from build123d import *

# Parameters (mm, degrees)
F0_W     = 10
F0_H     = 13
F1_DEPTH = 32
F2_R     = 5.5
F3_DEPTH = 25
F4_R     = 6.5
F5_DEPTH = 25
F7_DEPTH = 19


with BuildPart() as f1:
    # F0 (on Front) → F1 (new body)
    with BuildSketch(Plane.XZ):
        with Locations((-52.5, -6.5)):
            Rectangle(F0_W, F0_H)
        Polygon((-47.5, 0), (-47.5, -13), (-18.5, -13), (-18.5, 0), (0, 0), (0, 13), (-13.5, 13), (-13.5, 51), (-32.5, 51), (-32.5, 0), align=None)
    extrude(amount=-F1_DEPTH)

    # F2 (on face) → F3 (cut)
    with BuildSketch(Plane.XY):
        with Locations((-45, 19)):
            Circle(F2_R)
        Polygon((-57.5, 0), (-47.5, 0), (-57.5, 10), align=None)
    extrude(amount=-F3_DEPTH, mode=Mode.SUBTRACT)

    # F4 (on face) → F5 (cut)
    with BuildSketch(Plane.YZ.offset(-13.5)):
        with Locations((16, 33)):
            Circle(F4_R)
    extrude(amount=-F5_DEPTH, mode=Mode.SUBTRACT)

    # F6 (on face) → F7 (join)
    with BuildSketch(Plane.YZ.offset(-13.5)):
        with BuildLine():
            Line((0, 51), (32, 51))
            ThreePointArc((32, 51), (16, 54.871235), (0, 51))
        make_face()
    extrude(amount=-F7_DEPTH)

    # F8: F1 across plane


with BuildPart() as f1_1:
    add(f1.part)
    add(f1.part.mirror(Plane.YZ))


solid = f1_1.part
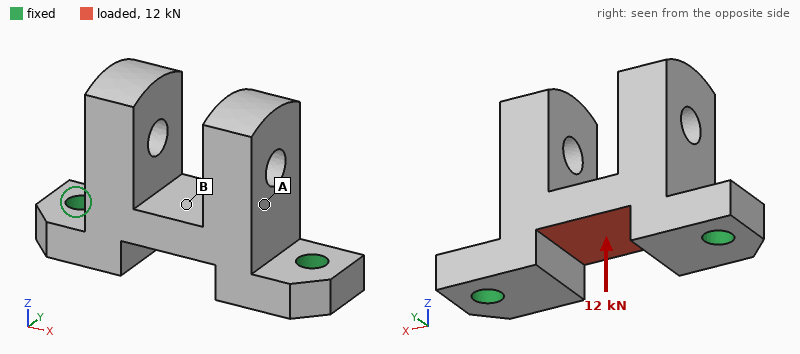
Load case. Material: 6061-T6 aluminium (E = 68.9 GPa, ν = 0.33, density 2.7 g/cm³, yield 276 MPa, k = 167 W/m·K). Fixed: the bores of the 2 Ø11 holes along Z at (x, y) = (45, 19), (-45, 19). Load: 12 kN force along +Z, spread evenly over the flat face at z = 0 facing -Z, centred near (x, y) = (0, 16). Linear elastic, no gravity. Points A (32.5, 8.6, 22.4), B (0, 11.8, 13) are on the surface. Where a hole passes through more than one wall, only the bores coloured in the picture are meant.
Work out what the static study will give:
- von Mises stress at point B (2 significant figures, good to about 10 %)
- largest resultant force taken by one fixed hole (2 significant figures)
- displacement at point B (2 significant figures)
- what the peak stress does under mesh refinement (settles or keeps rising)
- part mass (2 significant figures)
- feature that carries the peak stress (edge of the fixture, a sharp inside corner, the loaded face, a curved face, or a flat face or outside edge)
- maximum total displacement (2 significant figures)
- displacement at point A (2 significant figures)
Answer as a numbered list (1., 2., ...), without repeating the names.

1. 65 MPa
2. 9.4 kN
3. 52 µm
4. keeps rising
5. 270 g
6. edge of the fixture
7. 80 µm
8. 32 µm
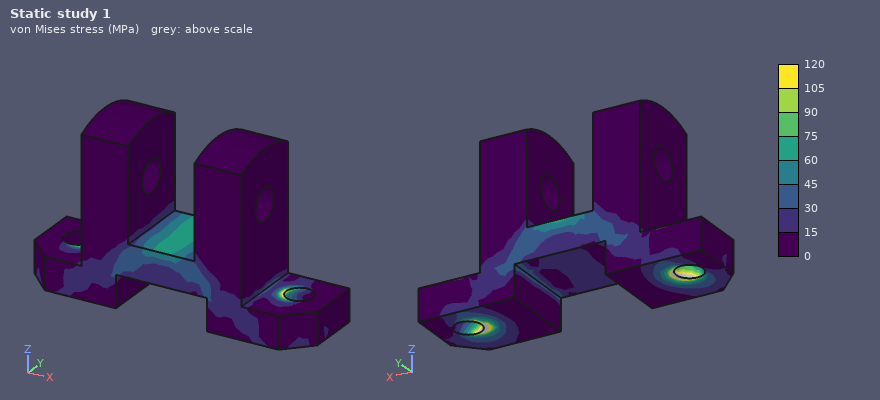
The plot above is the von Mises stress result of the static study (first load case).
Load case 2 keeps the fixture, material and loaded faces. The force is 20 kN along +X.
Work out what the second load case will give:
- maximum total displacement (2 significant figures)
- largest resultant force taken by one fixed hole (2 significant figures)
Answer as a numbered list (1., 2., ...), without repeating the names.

1. 49 µm
2. 10 kN
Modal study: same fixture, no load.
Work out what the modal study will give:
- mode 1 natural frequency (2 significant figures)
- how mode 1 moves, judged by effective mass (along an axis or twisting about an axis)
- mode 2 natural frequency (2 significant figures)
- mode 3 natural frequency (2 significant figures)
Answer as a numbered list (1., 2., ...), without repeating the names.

1. 2500 Hz
2. along Y
3. 3900 Hz
4. 4300 Hz
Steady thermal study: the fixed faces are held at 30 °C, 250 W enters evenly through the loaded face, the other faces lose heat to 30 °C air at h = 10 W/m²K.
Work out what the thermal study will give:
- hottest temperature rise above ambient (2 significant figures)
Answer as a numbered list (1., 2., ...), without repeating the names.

1. 66 K
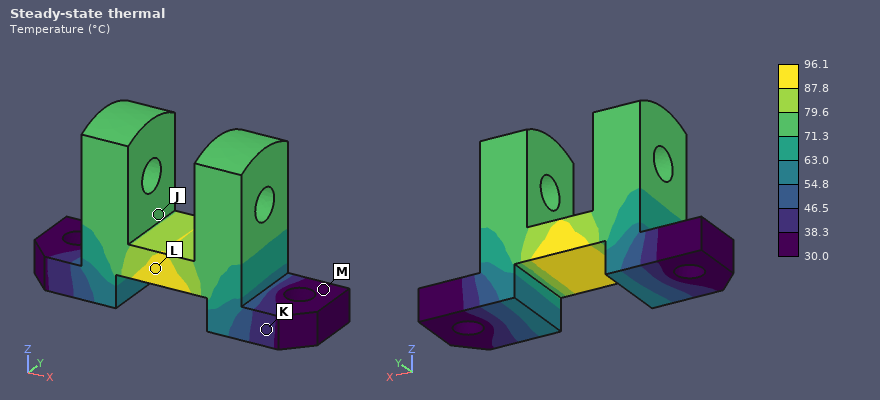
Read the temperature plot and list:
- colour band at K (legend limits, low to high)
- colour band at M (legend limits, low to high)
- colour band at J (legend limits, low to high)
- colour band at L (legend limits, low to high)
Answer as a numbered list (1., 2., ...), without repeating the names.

1. 38.3 to 46.5 °C
2. 30.0 to 38.3 °C
3. 71.3 to 79.6 °C
4. 87.8 to 96.1 °C
